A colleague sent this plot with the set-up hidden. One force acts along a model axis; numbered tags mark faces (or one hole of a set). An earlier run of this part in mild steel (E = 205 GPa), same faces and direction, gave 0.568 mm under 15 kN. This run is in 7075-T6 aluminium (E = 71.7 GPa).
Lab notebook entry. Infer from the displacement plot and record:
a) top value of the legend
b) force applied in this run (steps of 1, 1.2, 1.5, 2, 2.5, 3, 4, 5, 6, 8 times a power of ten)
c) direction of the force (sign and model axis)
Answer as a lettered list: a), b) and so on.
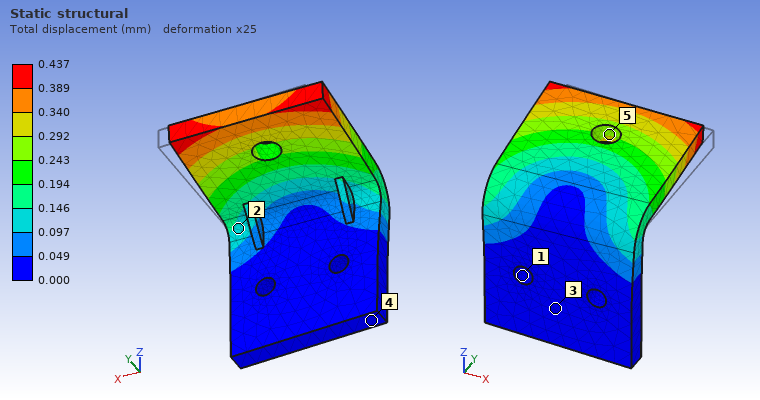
a) 0.437 mm
b) 4 kN
c) -X
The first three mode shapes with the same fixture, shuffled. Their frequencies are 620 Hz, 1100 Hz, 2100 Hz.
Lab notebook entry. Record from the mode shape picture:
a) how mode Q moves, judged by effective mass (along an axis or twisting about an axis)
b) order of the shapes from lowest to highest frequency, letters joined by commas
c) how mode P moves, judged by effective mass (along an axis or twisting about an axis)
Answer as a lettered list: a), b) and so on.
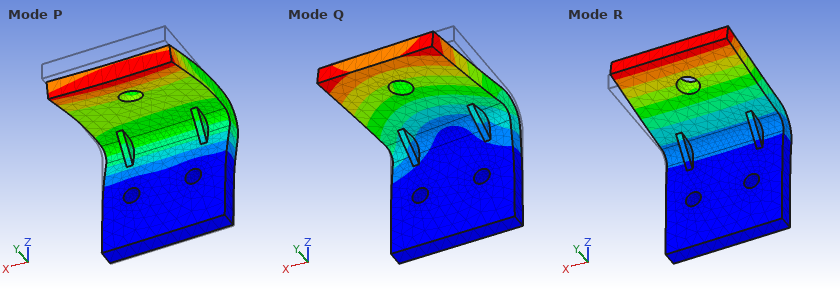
a) along X
b) R, Q, P
c) along Y
